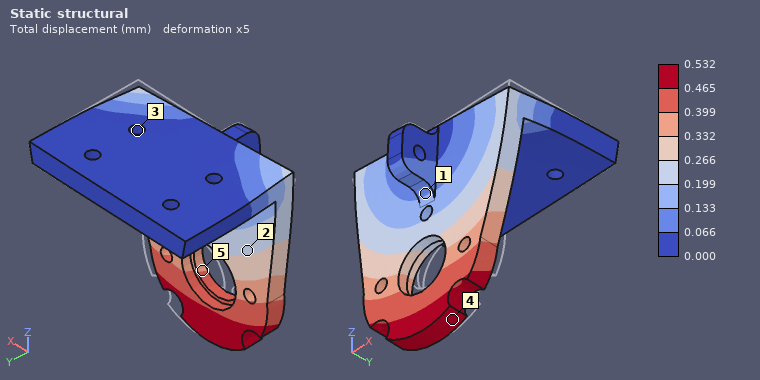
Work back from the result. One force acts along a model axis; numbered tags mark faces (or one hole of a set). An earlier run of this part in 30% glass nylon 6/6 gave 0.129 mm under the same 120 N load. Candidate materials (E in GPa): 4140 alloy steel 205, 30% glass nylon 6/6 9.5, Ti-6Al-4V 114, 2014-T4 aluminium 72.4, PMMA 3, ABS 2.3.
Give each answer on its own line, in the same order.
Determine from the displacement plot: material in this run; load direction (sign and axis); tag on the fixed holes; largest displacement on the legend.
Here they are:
ABS
-X
3
0.532 mm
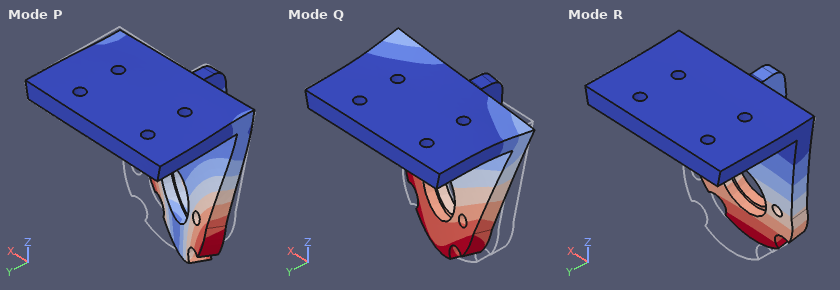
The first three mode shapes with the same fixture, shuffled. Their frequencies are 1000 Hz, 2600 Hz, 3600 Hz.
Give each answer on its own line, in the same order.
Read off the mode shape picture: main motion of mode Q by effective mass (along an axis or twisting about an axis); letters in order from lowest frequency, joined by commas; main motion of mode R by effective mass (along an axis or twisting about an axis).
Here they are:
along X
R, Q, P
along Y
